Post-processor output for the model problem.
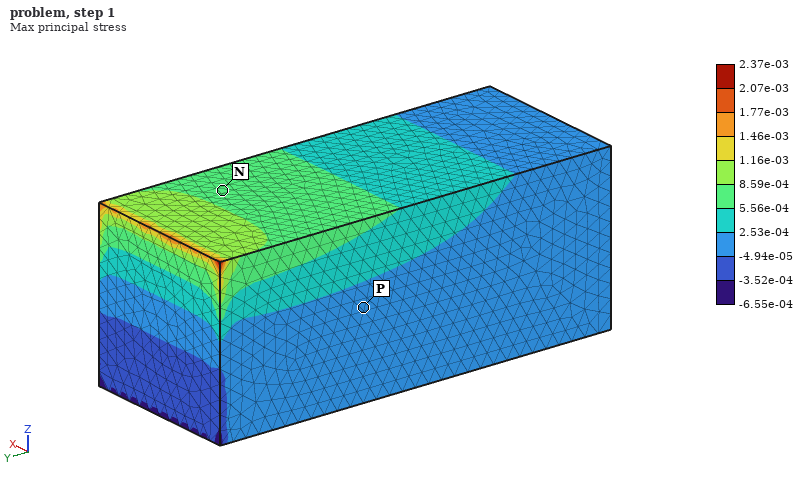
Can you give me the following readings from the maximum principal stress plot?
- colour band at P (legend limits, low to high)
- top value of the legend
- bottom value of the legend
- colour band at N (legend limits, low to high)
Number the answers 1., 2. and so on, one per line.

1. -4.94e-05 to 2.53e-04
2. 2.37e-03
3. -6.55e-04
4. 5.56e-04 to 8.59e-04
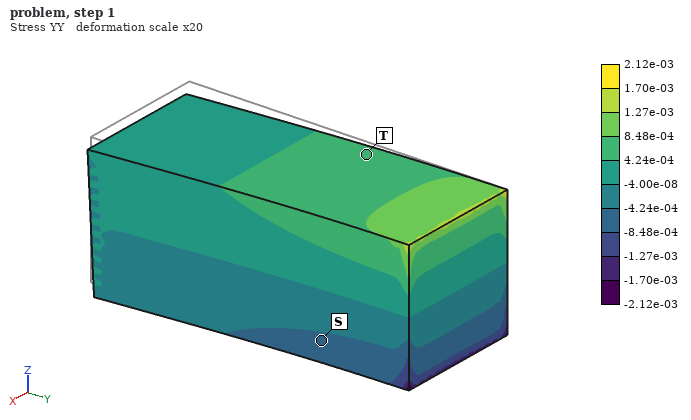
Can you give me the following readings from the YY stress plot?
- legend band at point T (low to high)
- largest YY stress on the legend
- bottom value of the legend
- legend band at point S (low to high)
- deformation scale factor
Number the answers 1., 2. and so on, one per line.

1. 4.24e-04 to 8.48e-04
2. 2.12e-03
3. -2.12e-03
4. -8.48e-04 to -4.24e-04
5. 20
